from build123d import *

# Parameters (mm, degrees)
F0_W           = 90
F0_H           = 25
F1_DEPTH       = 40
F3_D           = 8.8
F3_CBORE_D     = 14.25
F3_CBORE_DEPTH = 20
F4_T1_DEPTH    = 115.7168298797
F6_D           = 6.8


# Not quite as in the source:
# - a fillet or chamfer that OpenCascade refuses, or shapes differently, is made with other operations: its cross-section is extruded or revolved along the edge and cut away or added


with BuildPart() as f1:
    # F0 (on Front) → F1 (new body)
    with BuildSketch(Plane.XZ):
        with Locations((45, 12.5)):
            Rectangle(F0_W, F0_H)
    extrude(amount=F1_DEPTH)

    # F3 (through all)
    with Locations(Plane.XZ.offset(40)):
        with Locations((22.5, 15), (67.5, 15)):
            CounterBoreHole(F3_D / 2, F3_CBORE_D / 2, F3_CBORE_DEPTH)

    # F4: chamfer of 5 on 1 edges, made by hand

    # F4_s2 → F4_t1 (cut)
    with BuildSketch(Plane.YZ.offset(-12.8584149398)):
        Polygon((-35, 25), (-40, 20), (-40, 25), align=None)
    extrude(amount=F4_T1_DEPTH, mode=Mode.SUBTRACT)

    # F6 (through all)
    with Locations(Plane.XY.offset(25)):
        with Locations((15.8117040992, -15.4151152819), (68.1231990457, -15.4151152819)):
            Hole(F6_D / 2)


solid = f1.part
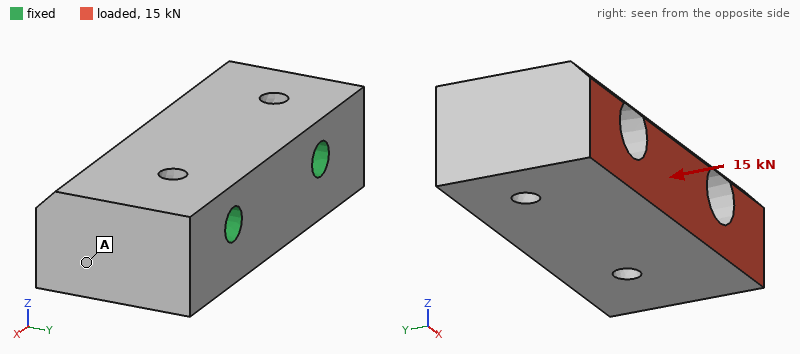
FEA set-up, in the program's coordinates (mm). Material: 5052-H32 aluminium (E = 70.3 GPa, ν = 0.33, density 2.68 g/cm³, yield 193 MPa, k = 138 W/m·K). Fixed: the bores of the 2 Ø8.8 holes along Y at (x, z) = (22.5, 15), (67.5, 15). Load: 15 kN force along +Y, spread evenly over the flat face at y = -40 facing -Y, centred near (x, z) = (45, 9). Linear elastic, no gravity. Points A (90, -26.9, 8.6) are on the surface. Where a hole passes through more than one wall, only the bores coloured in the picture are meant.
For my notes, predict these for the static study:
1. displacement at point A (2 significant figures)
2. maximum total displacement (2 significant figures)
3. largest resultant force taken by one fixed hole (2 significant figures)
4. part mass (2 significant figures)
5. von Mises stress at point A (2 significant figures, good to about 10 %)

9.9 µm
18 µm
7.6 kN
210 g
8.6 MPa
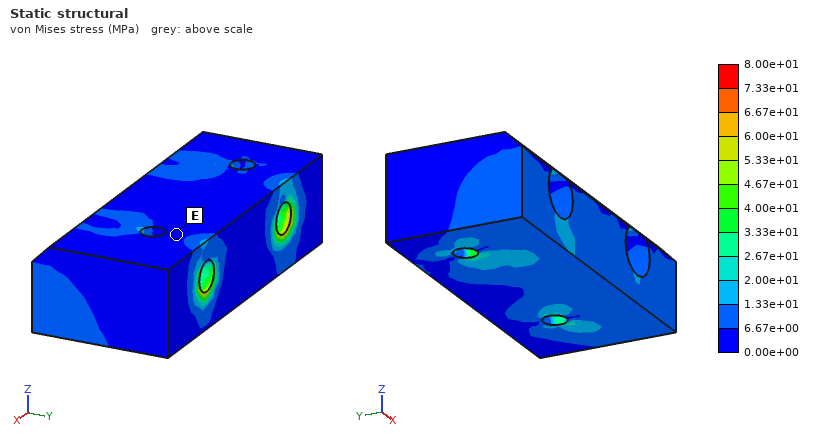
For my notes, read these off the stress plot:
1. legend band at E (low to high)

0.00e+00 to 6.67e+00 MPa
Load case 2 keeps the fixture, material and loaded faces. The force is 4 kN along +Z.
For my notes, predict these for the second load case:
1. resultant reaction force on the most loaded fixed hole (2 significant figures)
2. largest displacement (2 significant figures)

2.0 kN
20 µm
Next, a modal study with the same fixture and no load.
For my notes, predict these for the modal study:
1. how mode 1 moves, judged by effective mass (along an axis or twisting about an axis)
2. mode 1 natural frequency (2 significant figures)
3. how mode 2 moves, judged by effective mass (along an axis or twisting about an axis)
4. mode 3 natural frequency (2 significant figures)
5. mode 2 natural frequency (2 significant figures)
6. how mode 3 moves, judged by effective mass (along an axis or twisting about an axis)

along Z
10 kHz
twisting about Y
15 kHz
12 kHz
along X
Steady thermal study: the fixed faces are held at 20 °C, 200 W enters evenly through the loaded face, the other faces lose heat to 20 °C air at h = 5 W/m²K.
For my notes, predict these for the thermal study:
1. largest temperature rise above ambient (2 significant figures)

31 K
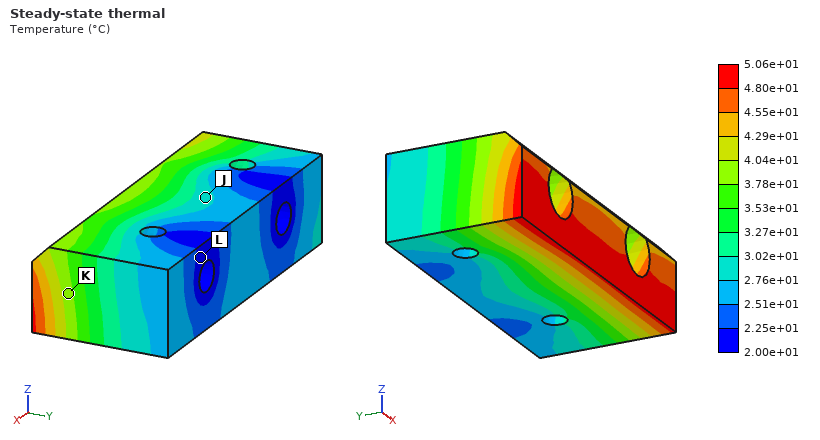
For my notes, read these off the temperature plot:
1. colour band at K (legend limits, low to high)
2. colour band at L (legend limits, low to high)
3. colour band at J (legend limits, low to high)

3.78e+01 to 4.04e+01 °C
2.00e+01 to 2.25e+01 °C
2.76e+01 to 3.02e+01 °C
